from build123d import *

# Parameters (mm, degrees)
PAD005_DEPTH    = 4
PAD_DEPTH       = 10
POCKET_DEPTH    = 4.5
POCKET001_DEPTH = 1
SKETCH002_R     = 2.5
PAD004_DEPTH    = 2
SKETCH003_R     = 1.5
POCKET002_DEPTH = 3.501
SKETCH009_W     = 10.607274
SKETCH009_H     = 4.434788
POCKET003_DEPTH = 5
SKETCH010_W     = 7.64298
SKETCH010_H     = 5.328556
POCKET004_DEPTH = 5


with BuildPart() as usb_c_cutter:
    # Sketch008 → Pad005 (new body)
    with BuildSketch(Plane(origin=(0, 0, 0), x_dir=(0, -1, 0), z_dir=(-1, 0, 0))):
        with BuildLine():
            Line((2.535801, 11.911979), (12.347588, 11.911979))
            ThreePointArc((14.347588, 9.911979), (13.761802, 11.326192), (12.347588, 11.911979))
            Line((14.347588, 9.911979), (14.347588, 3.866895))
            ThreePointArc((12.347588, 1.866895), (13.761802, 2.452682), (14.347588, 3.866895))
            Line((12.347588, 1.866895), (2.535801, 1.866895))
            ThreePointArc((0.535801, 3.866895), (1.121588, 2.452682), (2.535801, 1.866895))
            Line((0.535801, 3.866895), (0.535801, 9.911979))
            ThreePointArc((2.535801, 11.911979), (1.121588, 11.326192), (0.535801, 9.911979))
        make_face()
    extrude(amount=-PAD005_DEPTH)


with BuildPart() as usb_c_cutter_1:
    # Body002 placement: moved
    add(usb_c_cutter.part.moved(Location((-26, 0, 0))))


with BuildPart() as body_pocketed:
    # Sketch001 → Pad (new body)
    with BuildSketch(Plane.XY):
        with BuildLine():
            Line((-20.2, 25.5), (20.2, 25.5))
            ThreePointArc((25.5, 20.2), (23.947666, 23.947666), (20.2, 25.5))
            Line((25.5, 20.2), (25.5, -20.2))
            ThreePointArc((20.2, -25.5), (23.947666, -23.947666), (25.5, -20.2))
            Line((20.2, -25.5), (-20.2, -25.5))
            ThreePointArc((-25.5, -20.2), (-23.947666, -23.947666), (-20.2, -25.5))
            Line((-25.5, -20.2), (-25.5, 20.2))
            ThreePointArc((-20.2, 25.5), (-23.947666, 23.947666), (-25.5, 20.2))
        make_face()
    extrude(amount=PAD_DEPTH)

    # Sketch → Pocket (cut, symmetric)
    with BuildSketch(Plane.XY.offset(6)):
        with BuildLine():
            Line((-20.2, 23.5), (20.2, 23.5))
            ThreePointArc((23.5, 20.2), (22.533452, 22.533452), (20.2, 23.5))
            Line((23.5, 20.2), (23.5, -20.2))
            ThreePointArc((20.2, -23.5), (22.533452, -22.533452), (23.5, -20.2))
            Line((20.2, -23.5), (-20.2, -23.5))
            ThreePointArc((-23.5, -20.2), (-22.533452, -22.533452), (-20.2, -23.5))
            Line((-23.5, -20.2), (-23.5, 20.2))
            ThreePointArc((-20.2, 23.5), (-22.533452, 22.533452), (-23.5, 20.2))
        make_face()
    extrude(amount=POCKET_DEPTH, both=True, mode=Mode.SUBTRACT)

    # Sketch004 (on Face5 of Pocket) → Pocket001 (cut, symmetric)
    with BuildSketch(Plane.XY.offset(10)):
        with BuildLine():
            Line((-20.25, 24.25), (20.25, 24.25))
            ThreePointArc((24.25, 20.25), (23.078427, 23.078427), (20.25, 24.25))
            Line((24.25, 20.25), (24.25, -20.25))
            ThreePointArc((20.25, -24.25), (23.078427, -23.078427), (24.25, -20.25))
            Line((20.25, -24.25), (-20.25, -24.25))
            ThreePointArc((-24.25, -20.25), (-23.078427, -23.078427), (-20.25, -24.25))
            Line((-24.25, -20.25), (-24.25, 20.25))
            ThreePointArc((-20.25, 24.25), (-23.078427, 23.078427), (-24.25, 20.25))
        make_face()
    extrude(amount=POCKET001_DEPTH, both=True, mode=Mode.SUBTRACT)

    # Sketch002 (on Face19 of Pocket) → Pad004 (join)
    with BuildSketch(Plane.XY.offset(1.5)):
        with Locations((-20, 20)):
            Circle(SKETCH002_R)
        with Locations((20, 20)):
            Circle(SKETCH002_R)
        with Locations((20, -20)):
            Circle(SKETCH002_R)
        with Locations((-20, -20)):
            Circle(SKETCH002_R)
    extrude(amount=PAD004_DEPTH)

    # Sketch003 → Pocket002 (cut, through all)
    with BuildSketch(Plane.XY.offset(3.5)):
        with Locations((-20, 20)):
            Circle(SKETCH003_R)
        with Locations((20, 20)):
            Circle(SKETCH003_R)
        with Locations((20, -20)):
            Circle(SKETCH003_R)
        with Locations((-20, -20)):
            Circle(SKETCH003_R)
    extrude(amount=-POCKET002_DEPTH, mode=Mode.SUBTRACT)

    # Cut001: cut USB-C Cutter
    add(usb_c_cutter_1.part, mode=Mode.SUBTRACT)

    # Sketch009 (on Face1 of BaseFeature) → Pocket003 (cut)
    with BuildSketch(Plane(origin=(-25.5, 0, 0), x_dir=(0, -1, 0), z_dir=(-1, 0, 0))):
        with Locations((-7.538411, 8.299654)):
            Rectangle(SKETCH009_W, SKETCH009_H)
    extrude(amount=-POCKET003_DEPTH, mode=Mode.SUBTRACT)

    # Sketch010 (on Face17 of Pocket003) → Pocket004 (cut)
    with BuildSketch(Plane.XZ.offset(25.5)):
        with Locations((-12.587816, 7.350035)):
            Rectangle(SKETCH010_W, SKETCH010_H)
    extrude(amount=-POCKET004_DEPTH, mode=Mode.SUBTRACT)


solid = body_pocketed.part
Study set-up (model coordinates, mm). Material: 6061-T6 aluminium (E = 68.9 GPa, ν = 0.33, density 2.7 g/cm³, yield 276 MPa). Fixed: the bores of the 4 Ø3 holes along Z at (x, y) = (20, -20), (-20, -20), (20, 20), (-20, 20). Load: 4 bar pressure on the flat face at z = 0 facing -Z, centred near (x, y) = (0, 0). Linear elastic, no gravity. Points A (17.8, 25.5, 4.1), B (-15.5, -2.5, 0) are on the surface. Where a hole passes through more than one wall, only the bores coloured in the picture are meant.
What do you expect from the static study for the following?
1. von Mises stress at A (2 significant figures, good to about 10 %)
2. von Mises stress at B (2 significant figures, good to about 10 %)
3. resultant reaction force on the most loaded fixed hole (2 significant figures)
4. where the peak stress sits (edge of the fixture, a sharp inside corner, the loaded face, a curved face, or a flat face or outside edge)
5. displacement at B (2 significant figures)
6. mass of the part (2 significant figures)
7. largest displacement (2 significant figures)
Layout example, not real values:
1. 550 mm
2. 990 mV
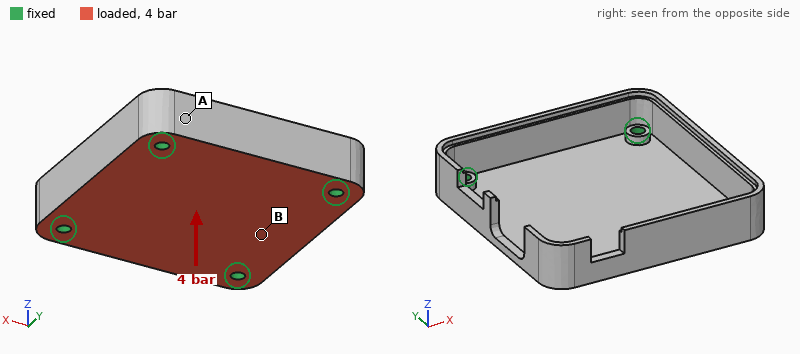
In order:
1. 24 MPa
2. 56 MPa
3. 270 N
4. the loaded face
5. 0.12 mm
6. 18 g
7. 0.20 mm
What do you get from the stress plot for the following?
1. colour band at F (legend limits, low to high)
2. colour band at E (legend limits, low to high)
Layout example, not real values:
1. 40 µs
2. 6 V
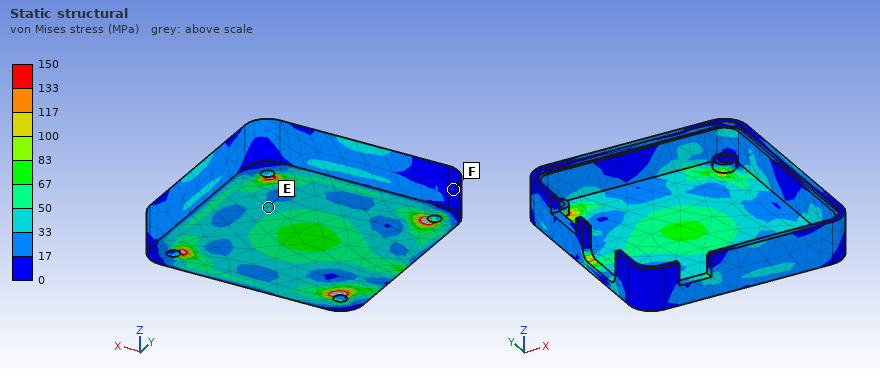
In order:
1. 0 to 17 MPa
2. 33 to 50 MPa
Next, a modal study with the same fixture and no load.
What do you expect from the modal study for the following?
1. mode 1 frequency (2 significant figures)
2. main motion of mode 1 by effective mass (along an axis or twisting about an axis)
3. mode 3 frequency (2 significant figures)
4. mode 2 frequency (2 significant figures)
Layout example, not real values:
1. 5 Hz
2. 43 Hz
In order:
1. 4400 Hz
2. along Z
3. 8800 Hz
4. 7300 Hz
